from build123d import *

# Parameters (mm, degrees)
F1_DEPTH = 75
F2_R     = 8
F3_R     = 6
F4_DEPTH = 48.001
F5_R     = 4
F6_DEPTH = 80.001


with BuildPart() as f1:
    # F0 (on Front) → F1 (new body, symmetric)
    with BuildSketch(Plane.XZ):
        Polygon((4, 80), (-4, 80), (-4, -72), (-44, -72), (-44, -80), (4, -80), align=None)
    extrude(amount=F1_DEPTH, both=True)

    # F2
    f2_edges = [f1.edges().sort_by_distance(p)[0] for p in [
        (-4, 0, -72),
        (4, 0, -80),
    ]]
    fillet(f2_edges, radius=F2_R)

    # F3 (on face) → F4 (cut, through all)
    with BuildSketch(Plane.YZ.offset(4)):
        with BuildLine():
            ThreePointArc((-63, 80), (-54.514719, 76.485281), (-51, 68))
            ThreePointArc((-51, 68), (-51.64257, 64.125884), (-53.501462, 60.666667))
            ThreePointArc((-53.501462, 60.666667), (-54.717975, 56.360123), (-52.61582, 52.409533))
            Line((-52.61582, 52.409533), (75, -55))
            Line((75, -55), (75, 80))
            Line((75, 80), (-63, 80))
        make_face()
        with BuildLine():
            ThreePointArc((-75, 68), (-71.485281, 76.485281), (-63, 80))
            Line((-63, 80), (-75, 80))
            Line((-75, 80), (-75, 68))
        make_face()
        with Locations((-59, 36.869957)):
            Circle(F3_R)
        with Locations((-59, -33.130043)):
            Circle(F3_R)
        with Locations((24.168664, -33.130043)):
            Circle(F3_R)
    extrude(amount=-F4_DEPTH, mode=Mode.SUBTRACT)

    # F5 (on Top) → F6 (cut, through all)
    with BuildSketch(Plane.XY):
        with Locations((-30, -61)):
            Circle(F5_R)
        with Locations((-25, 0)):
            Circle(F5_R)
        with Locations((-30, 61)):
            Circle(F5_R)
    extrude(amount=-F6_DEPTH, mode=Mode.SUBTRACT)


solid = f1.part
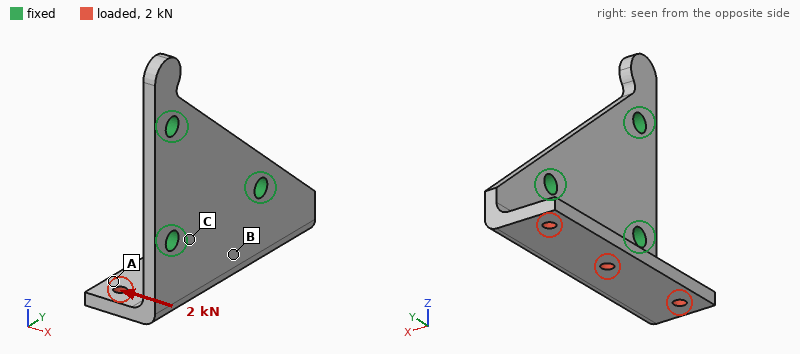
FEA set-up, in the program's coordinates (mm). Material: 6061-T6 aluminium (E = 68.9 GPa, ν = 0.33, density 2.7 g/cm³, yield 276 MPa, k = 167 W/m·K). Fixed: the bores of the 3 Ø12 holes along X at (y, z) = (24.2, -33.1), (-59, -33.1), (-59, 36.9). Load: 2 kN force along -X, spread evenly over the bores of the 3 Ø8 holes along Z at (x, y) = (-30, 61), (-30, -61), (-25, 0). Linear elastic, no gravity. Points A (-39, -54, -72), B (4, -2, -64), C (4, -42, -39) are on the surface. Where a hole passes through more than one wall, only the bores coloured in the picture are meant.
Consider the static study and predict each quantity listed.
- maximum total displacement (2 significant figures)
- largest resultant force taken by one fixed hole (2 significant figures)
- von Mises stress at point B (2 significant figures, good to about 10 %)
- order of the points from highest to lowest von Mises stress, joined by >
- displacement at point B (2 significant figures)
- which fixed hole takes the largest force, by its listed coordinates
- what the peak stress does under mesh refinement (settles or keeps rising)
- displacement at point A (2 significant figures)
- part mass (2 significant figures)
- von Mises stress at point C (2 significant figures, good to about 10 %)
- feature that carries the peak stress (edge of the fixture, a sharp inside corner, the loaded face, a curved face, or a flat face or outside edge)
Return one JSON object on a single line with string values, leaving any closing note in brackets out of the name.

{"maximum total displacement": "0.30 mm", "largest resultant force taken by one fixed hole": "1.4 kN", "von Mises stress at point B": "18 MPa", "order of the points from highest to lowest von Mises stress, joined by >": "C > B > A", "displacement at point B": "0.090 mm", "which fixed hole takes the largest force, by its listed coordinates": "(24.2, -33.1)", "what the peak stress does under mesh refinement": "keeps rising", "displacement at point A": "0.19 mm", "part mass": "410 g", "von Mises stress at point C": "30 MPa", "feature that carries the peak stress": "edge of the fixture"}
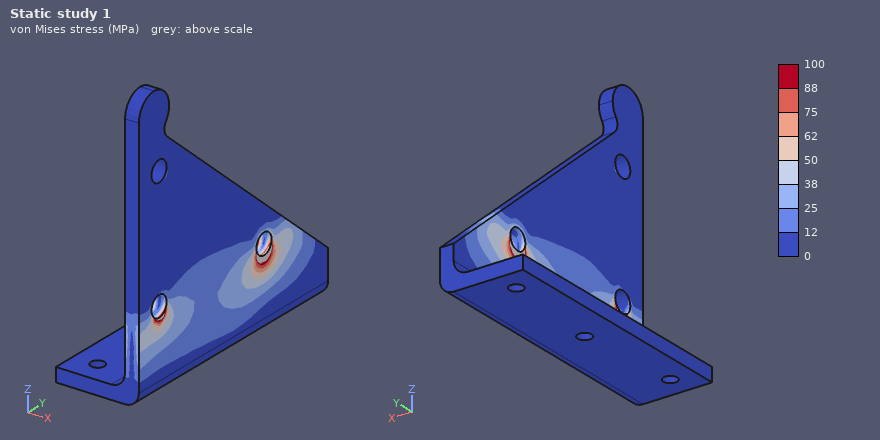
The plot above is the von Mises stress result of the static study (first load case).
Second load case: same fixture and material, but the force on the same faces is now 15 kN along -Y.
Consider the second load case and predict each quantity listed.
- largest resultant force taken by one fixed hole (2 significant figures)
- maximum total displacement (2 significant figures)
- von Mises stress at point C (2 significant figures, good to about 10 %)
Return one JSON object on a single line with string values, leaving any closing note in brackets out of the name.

{"largest resultant force taken by one fixed hole": "11 kN", "maximum total displacement": "0.89 mm", "von Mises stress at point C": "61 MPa"}
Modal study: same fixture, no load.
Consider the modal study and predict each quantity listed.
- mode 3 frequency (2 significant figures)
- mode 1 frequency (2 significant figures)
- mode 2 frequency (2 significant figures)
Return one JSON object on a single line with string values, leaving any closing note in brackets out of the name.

{"mode 3 frequency": "3300 Hz", "mode 1 frequency": "1100 Hz", "mode 2 frequency": "1700 Hz"}
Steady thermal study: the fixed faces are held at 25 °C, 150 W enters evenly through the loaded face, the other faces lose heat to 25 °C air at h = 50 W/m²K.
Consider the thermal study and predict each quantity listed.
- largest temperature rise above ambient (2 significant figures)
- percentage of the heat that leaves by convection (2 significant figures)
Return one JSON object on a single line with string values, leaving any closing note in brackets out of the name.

{"largest temperature rise above ambient": "59 K", "percentage of the heat that leaves by convection": "28 %"}
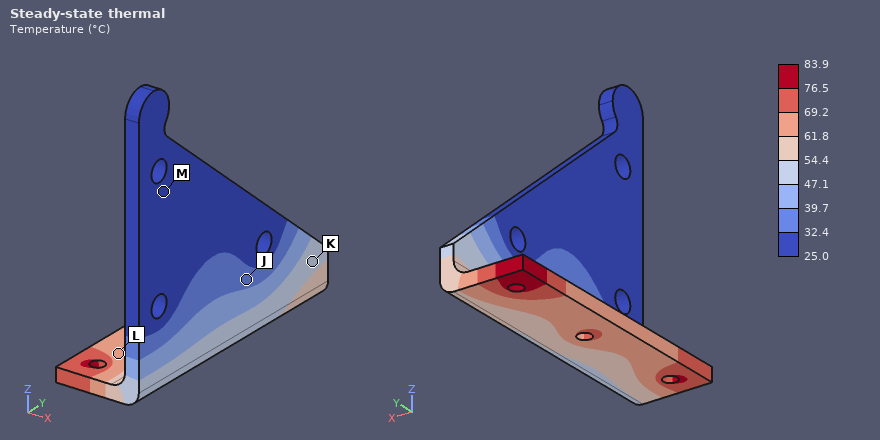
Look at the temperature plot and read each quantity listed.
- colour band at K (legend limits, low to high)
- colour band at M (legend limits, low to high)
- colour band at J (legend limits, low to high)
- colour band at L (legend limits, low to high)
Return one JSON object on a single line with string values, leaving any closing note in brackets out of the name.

{"colour band at K": "47.1 to 54.4 °C", "colour band at M": "25.0 to 32.4 °C", "colour band at J": "32.4 to 39.7 °C", "colour band at L": "61.8 to 69.2 °C"}
